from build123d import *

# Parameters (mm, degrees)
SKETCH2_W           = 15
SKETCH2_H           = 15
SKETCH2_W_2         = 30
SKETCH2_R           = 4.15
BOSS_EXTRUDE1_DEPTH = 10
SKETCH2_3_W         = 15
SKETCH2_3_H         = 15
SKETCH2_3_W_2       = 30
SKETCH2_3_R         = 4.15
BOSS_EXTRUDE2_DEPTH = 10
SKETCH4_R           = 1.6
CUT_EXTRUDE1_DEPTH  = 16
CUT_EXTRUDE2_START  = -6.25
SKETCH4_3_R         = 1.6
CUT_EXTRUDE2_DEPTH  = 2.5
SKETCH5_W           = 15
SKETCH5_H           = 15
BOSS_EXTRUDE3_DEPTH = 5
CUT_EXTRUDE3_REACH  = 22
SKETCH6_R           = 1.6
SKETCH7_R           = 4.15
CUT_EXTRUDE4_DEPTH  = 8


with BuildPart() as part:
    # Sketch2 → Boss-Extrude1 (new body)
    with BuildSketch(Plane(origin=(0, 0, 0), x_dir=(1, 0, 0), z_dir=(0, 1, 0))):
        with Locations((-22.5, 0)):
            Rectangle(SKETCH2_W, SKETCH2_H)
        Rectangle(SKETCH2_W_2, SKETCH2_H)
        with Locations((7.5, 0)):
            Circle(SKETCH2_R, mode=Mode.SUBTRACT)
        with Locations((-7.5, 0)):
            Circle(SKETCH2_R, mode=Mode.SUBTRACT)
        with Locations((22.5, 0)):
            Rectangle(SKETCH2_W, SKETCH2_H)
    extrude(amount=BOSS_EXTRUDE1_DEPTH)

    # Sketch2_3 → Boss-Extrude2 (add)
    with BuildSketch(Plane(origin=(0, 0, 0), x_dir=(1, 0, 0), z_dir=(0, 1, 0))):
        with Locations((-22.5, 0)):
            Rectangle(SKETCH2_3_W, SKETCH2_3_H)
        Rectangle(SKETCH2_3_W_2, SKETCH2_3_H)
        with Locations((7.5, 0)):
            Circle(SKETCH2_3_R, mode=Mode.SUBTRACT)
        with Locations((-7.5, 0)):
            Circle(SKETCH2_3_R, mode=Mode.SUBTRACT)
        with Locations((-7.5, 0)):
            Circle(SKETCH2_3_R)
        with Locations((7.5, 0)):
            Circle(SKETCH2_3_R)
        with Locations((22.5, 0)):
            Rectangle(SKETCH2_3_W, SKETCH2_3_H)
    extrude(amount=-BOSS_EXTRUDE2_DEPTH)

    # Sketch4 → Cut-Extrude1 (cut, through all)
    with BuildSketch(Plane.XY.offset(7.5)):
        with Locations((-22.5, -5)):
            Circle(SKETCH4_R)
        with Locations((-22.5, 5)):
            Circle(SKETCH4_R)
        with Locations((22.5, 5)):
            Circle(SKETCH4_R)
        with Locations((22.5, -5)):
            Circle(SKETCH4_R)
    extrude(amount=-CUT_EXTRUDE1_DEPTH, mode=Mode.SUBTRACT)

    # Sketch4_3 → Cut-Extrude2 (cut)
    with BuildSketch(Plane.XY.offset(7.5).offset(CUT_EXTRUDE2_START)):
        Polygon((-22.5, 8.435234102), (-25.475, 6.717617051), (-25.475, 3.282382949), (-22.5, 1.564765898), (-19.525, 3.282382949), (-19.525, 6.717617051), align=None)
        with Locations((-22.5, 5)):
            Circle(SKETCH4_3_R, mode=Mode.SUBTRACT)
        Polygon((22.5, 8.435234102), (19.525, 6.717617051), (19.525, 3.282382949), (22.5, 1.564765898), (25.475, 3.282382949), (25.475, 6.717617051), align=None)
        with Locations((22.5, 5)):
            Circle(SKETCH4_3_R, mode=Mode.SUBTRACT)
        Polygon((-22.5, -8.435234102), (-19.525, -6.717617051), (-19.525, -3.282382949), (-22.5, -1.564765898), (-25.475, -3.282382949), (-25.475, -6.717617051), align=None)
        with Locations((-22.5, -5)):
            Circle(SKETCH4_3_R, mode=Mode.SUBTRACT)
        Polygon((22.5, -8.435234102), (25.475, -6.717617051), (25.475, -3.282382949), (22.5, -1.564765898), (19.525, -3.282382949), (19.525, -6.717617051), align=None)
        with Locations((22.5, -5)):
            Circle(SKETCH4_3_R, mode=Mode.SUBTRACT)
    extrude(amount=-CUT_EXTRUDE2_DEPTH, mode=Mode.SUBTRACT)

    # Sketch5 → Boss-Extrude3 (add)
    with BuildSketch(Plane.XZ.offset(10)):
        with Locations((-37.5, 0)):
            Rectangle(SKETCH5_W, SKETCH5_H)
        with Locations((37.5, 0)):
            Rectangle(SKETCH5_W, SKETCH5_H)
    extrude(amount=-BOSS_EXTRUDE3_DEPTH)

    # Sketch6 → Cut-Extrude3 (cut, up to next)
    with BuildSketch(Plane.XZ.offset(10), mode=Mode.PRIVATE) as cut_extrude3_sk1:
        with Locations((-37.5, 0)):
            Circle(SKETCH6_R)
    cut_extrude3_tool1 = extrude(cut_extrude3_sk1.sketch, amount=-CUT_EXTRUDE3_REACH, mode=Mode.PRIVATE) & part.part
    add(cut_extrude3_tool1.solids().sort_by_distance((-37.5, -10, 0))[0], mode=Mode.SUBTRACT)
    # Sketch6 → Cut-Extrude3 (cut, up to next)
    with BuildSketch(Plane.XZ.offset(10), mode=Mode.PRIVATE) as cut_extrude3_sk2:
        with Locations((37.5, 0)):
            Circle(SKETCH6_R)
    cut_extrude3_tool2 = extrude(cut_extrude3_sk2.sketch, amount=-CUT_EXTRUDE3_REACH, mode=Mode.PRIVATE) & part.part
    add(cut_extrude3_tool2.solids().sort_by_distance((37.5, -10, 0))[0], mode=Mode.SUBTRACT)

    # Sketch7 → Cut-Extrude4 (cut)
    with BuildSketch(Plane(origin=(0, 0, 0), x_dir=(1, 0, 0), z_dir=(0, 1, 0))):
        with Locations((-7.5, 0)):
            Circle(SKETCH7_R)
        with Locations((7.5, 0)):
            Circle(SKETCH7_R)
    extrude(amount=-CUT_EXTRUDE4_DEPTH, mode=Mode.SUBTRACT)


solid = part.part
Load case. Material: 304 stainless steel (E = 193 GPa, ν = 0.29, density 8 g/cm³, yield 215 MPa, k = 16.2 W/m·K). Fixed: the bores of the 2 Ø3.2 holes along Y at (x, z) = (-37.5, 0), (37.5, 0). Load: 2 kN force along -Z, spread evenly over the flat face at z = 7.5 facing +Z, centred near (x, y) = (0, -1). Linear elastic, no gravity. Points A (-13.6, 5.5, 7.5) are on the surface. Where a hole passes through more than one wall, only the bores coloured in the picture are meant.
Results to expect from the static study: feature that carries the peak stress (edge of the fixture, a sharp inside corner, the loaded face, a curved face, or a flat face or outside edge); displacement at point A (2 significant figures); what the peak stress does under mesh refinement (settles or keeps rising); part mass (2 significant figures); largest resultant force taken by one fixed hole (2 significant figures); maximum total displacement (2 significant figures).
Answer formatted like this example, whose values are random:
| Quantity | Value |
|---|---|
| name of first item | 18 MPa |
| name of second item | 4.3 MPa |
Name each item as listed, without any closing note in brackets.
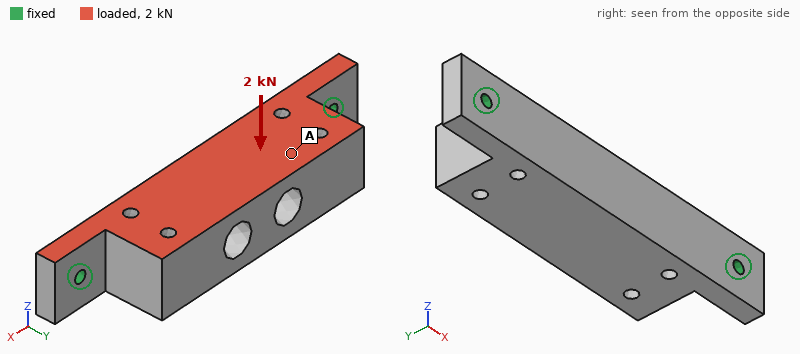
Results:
| Quantity | Value |
|---|---|
| feature that carries the peak stress | edge of the fixture |
| displacement at point A | 31 µm |
| what the peak stress does under mesh refinement | keeps rising |
| part mass | 140 g |
| largest resultant force taken by one fixed hole | 1.0 kN |
| maximum total displacement | 39 µm |
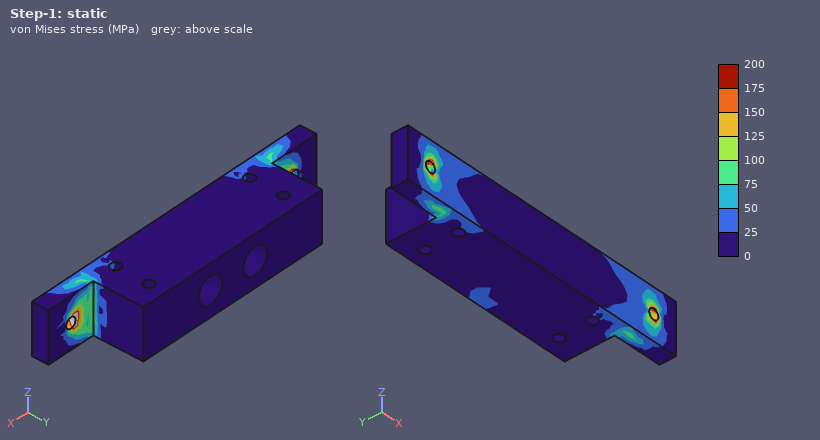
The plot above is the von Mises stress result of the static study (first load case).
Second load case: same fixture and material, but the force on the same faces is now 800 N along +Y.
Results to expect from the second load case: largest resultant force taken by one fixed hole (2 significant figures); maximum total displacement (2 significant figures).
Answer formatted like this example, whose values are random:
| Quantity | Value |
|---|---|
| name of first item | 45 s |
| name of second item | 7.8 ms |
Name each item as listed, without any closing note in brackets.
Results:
| Quantity | Value |
|---|---|
| largest resultant force taken by one fixed hole | 490 N |
| maximum total displacement | 14 µm |
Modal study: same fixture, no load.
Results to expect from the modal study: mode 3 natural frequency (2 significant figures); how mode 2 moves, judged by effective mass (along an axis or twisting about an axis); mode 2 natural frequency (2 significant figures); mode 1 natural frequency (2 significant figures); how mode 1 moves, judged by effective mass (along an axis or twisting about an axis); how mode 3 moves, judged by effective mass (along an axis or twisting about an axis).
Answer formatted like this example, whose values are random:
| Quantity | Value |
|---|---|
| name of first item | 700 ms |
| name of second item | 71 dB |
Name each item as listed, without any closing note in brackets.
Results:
| Quantity | Value |
|---|---|
| mode 3 natural frequency | 9100 Hz |
| how mode 2 moves, judged by effective mass | along Y |
| mode 2 natural frequency | 7000 Hz |
| mode 1 natural frequency | 3700 Hz |
| how mode 1 moves, judged by effective mass | along Z |
| how mode 3 moves, judged by effective mass | along Z |
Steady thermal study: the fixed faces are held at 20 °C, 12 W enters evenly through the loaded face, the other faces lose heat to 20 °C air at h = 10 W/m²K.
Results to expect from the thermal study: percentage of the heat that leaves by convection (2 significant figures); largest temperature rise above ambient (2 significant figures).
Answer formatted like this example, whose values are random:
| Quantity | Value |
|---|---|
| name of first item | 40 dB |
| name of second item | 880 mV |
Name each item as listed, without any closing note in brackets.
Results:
| Quantity | Value |
|---|---|
| percentage of the heat that leaves by convection | 22 % |
| largest temperature rise above ambient | 60 K |
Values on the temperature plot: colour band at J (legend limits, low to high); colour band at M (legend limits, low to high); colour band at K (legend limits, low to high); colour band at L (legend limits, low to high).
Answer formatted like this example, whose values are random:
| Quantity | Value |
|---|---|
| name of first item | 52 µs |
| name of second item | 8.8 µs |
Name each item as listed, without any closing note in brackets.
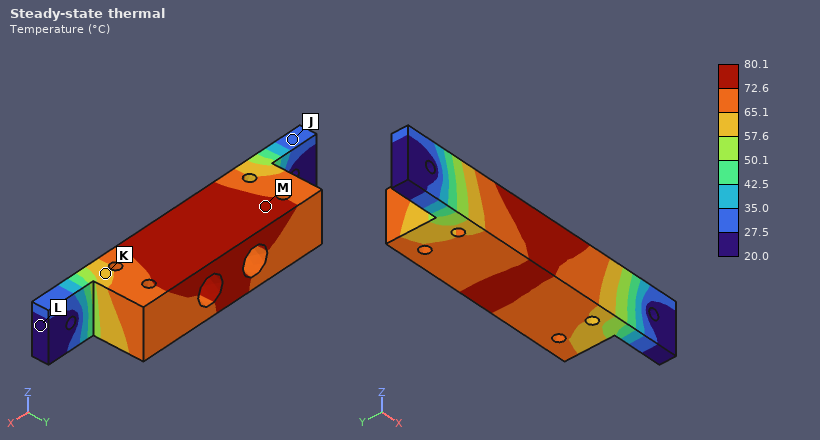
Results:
| Quantity | Value |
|---|---|
| colour band at J | 27.5 to 35.0 °C |
| colour band at M | 72.6 to 80.1 °C |
| colour band at K | 57.6 to 65.1 °C |
| colour band at L | 20.0 to 27.5 °C |
